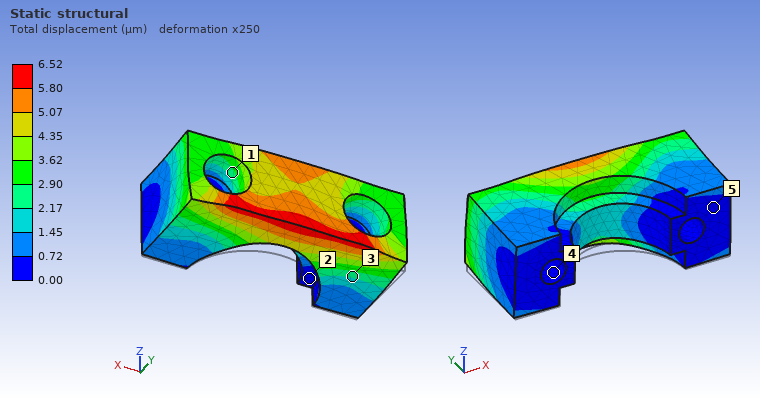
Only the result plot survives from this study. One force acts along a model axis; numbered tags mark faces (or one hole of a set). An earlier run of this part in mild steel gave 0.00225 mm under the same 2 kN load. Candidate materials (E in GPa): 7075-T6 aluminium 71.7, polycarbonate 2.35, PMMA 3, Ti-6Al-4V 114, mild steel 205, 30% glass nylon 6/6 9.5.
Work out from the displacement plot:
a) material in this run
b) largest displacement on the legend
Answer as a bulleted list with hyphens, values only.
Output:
- 7075-T6 aluminium
- 6.52 µm
